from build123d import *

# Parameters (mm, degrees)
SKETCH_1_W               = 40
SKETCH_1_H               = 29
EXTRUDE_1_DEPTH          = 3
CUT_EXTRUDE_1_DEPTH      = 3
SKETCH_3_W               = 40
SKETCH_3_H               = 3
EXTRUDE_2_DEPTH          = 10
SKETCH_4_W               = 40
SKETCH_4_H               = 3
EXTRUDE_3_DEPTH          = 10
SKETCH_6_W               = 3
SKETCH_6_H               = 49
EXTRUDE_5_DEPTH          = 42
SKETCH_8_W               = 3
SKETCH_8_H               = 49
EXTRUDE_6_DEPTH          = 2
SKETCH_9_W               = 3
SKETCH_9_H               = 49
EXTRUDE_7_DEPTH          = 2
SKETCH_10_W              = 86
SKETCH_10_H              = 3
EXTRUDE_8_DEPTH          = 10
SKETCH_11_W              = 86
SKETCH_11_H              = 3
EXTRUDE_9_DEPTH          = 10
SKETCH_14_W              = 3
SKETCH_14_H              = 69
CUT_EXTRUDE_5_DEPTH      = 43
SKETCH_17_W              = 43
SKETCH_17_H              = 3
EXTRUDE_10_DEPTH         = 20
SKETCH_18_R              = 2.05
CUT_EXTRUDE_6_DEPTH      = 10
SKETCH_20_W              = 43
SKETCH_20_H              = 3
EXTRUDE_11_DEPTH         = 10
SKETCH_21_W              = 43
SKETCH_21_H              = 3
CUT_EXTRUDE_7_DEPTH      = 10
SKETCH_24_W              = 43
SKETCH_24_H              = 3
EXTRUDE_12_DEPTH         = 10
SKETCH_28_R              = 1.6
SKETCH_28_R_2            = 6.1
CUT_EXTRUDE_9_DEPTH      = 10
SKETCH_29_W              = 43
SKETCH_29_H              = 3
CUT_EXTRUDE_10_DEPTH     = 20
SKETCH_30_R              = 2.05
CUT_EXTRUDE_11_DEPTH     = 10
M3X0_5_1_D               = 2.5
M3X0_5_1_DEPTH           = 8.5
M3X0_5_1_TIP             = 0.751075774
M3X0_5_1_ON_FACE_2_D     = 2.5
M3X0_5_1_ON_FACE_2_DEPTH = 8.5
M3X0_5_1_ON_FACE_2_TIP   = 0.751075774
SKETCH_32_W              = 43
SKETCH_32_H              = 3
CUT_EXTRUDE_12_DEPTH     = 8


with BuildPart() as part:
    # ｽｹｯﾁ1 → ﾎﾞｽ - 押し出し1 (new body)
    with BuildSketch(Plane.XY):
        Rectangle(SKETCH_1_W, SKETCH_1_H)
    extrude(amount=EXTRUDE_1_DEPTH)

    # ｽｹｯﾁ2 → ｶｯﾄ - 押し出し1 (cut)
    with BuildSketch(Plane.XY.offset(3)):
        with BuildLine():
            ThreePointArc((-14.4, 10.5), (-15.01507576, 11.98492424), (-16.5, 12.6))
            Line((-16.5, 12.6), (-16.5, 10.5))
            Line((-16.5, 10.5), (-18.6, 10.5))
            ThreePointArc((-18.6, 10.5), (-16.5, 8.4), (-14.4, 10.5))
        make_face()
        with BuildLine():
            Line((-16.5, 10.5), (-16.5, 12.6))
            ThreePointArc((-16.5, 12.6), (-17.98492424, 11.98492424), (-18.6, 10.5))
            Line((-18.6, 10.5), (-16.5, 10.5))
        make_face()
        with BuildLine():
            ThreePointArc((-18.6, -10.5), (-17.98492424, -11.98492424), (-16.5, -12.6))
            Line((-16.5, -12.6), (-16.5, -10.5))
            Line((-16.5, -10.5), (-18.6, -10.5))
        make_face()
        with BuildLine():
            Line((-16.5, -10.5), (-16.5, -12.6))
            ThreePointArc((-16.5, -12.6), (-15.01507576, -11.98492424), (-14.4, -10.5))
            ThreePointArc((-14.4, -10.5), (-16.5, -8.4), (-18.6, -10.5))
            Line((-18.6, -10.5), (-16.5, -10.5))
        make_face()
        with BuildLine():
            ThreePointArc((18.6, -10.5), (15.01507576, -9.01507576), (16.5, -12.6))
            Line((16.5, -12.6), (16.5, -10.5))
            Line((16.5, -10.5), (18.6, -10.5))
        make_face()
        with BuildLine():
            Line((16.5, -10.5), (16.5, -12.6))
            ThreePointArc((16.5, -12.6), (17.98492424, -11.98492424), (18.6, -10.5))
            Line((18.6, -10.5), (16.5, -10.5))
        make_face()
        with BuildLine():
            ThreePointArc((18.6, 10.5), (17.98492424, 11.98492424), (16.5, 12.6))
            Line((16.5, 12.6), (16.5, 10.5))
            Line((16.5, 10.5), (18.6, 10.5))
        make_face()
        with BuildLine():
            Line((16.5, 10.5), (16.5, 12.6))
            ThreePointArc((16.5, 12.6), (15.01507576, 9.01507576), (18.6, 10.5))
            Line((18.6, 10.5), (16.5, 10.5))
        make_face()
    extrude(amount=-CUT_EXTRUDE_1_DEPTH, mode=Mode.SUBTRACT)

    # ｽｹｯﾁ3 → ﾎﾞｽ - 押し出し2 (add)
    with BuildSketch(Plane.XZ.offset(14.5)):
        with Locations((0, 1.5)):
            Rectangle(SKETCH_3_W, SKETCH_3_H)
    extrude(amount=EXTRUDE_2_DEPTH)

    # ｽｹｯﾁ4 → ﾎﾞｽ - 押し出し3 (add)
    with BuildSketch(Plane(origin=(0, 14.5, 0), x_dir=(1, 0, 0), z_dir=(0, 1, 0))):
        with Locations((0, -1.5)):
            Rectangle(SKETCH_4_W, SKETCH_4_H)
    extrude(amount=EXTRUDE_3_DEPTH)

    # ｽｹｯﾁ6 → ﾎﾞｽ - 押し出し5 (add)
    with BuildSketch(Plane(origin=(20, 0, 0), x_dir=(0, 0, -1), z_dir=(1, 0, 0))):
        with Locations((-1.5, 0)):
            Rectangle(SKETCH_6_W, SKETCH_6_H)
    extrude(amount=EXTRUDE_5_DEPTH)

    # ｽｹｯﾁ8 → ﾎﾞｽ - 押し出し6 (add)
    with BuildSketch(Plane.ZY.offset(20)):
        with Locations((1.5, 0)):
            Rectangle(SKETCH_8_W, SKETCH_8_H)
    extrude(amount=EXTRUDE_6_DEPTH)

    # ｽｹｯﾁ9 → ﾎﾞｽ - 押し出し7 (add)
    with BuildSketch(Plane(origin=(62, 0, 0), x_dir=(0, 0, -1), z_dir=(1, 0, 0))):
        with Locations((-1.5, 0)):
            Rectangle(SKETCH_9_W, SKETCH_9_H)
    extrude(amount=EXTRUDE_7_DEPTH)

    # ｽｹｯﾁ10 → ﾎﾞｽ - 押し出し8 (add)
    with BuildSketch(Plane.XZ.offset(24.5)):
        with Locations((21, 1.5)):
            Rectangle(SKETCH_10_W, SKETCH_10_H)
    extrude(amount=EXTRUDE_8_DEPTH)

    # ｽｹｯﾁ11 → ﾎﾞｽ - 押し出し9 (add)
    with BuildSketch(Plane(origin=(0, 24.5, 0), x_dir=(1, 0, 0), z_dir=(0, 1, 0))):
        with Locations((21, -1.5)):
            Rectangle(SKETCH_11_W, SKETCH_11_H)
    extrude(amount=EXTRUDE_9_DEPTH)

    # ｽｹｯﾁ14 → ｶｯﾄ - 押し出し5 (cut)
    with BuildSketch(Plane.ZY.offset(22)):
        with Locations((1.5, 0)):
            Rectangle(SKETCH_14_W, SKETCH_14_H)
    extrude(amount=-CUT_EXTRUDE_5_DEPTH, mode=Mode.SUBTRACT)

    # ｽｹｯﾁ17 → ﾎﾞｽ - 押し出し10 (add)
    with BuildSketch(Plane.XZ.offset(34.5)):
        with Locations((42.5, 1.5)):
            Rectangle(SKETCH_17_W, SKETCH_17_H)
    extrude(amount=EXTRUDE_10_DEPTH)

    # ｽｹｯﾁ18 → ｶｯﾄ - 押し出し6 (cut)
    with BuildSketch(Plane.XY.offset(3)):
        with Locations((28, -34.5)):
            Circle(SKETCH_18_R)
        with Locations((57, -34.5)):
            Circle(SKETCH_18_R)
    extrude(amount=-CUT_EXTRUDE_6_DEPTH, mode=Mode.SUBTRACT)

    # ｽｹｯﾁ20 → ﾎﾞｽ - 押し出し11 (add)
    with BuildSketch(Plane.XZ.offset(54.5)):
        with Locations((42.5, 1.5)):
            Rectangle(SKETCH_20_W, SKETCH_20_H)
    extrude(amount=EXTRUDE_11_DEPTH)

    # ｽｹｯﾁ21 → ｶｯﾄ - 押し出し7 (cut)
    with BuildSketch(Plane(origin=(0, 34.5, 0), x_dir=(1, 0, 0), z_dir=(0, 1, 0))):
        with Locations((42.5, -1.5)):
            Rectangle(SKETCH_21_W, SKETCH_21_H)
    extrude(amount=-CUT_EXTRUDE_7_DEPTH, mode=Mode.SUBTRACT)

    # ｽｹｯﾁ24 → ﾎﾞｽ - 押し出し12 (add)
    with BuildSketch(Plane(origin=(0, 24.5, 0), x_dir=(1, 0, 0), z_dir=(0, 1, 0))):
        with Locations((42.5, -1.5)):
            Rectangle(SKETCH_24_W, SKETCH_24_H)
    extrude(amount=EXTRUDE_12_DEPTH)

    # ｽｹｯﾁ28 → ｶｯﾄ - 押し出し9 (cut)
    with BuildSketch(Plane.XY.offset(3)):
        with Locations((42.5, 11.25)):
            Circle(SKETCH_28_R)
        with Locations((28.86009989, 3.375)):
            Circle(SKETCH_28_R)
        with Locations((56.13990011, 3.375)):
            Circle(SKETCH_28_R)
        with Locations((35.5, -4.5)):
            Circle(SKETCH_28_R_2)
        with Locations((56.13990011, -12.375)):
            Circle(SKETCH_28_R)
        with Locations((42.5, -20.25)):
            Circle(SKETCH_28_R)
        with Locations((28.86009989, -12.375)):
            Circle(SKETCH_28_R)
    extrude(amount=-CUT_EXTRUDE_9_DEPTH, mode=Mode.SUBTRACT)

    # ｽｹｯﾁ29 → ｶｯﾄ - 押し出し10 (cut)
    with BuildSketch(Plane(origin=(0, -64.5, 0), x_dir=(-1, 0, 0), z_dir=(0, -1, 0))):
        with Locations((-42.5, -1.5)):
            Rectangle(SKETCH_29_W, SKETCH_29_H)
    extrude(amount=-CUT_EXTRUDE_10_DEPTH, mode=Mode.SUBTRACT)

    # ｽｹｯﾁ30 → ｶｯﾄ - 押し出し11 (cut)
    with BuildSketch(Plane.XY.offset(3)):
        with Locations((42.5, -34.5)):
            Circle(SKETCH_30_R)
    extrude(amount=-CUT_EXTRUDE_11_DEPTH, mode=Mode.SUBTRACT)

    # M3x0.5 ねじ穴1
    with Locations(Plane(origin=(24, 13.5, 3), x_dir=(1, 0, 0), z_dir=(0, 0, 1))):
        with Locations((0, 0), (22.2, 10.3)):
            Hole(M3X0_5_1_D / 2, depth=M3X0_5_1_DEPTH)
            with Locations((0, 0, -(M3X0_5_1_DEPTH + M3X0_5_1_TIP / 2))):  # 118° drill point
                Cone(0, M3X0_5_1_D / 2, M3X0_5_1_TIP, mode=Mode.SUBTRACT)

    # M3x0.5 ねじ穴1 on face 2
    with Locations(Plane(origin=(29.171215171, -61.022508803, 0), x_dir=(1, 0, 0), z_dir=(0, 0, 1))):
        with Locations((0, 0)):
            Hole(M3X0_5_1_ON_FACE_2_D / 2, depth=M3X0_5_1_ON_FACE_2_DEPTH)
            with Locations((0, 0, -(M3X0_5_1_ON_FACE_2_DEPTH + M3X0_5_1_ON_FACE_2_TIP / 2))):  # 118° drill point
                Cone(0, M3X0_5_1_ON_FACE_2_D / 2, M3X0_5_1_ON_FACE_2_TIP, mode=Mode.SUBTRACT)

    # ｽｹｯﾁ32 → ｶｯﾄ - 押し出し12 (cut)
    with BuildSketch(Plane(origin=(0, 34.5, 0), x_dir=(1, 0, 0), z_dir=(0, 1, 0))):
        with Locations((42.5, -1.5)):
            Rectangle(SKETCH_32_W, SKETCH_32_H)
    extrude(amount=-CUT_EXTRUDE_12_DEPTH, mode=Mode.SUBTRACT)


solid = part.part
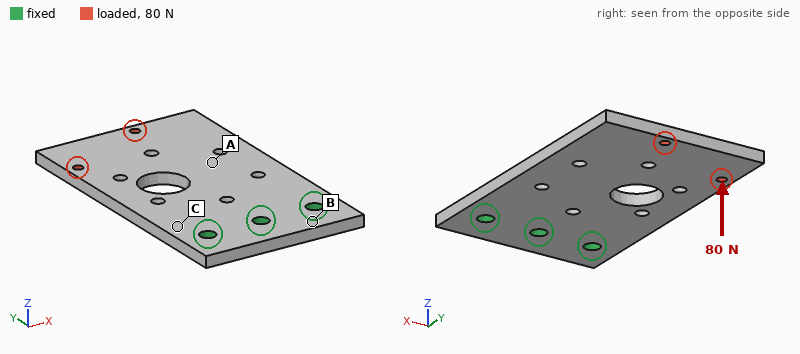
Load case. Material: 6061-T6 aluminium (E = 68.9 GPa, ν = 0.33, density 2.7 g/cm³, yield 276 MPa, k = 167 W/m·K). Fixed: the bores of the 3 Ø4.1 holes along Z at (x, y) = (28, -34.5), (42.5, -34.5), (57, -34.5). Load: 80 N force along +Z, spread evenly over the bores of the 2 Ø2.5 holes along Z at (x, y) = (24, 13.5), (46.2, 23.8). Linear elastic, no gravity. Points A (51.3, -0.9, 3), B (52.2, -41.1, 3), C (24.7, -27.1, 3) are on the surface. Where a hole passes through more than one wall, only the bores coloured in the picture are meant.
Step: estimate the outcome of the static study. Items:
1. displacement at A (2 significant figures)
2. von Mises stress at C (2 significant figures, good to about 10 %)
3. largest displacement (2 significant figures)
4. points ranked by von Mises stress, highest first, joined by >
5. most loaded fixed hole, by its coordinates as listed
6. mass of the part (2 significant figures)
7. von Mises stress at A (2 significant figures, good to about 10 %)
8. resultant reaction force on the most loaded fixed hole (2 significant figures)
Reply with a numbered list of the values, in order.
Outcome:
1. 0.26 mm
2. 58 MPa
3. 0.80 mm
4. C > A > B
5. (42.5, -34.5)
6. 23 g
7. 34 MPa
8. 60 N
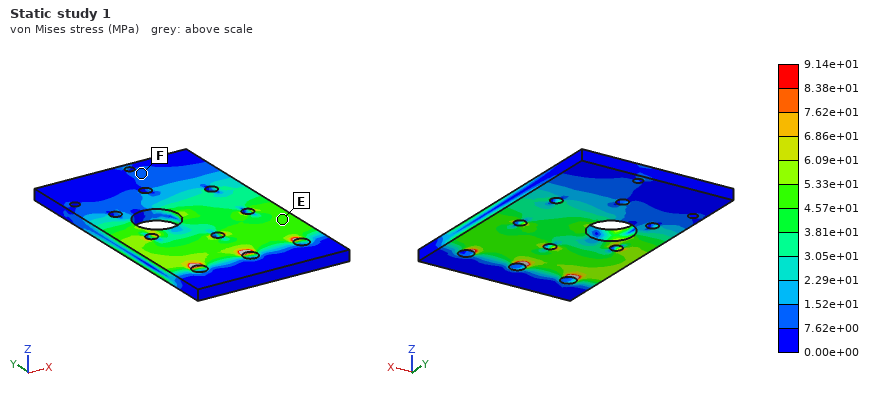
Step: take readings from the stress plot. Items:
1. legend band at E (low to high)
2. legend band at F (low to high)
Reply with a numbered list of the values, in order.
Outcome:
1. 4.57e+01 to 5.33e+01 MPa
2. 7.62e+00 to 1.52e+01 MPa
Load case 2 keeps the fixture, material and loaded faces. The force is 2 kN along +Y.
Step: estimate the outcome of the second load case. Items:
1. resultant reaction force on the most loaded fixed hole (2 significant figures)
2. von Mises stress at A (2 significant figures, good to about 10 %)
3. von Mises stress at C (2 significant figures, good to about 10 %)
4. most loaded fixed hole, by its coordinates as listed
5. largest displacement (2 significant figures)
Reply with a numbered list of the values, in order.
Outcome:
1. 1.2 kN
2. 14 MPa
3. 33 MPa
4. (28, -34.5)
5. 41 µm
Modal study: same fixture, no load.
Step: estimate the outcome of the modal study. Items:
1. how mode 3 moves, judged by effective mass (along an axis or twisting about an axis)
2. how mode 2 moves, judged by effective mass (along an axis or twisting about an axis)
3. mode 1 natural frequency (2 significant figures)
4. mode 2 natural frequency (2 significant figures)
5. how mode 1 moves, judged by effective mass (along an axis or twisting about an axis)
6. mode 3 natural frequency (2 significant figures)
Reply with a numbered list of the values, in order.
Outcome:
1. along Z
2. twisting about Y
3. 680 Hz
4. 2000 Hz
5. along Z
6. 4100 Hz
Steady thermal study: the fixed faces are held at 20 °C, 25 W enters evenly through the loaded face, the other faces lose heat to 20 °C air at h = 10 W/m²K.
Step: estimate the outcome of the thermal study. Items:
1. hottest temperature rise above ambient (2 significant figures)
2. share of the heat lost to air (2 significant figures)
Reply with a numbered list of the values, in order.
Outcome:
1. 77 K
2. 8.5 %
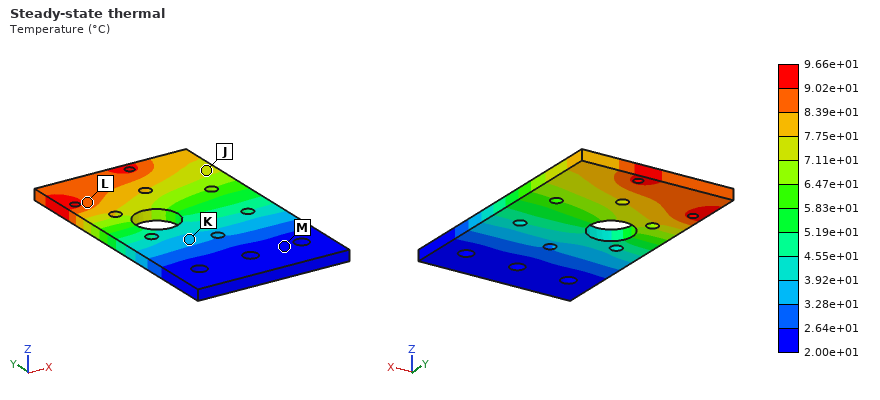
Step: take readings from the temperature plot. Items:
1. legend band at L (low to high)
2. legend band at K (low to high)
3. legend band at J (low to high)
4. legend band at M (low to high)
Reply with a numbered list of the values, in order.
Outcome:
1. 8.39e+01 to 9.02e+01 °C
2. 3.28e+01 to 3.92e+01 °C
3. 7.11e+01 to 7.75e+01 °C
4. 2.00e+01 to 2.64e+01 °C
